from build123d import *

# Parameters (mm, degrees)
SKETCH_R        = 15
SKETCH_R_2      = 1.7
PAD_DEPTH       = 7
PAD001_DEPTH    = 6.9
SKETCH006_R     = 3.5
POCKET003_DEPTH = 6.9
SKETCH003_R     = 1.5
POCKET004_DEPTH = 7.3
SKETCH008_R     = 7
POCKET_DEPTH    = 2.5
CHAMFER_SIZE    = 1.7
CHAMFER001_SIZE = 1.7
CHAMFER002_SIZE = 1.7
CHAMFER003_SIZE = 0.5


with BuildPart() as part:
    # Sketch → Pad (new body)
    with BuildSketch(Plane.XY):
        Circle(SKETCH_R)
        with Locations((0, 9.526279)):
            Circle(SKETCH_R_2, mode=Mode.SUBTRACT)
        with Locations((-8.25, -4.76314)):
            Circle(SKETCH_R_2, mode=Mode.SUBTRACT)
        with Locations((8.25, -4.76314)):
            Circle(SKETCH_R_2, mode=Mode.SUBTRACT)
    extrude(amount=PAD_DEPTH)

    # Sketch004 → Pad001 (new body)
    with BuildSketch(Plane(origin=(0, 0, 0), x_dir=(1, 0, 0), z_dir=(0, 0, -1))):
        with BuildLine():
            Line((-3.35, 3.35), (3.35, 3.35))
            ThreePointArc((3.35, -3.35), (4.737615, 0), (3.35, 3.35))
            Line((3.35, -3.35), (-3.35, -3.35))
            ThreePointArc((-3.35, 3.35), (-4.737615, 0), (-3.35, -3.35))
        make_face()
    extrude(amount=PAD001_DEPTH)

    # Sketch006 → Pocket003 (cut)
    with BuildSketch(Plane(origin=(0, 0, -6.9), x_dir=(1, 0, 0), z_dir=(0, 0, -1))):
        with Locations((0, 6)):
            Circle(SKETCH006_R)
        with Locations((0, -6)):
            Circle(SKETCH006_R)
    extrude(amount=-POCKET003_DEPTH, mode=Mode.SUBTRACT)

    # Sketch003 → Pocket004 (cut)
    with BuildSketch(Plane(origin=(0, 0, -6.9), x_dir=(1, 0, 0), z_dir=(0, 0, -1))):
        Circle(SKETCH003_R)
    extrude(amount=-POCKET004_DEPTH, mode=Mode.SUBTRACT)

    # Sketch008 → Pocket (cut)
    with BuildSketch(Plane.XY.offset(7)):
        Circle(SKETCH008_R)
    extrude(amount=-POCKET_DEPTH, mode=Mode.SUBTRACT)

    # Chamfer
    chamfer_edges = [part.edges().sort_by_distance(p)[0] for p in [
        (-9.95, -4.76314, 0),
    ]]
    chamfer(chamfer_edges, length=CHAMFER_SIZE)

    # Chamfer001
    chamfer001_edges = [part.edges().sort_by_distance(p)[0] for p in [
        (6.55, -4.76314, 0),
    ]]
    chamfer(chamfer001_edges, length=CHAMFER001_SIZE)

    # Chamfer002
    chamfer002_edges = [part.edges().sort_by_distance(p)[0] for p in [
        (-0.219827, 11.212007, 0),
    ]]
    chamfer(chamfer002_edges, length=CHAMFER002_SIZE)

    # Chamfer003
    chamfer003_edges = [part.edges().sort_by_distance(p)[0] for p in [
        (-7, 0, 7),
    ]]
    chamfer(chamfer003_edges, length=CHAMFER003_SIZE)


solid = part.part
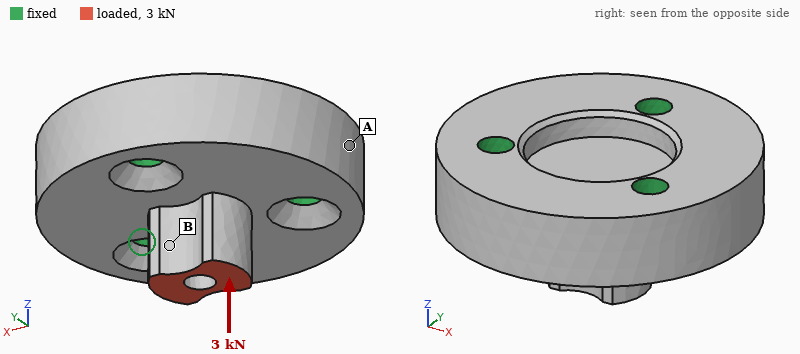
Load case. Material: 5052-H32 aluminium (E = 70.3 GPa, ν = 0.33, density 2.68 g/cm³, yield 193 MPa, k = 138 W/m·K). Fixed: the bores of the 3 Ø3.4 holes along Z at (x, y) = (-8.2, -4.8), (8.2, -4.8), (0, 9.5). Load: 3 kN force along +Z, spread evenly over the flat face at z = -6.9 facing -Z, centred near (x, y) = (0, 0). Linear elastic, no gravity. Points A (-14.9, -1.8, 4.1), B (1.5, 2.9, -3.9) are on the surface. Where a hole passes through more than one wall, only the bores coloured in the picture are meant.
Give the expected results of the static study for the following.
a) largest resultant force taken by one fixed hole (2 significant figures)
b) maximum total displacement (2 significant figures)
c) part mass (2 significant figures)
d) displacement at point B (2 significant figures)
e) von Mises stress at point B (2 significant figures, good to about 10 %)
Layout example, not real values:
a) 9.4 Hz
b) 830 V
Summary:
a) 1.1 kN
b) 15 µm
c) 12 g
d) 12 µm
e) 60 MPa
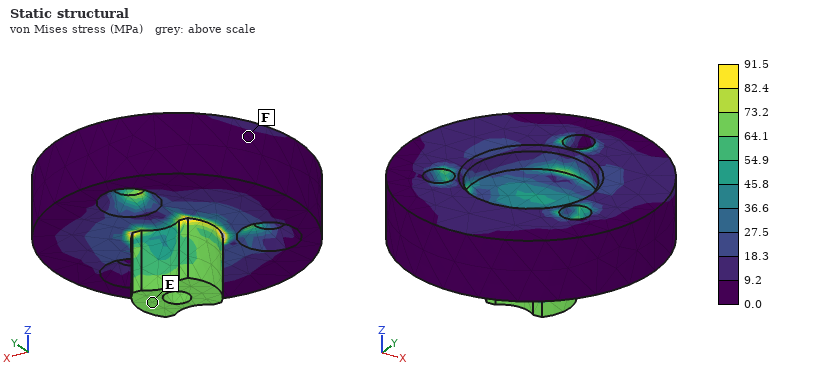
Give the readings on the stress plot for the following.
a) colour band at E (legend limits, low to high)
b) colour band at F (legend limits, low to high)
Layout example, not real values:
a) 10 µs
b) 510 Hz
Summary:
a) 64.1 to 73.2 MPa
b) 0.0 to 9.2 MPa
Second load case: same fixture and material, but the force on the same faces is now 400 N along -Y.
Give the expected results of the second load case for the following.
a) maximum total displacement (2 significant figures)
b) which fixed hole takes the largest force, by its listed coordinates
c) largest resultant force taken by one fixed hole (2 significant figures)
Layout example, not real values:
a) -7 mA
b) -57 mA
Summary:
a) 14 µm
b) (0, 9.5)
c) 320 N
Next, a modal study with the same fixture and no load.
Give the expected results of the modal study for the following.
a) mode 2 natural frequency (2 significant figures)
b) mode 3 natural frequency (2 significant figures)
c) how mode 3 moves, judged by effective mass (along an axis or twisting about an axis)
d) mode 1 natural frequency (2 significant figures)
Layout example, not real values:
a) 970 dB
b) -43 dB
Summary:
a) 38 kHz
b) 44 kHz
c) along Z
d) 38 kHz
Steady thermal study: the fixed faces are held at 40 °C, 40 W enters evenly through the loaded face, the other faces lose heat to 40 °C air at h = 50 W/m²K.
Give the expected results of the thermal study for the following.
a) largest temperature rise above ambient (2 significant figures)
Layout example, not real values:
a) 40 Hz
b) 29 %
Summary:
a) 61 K
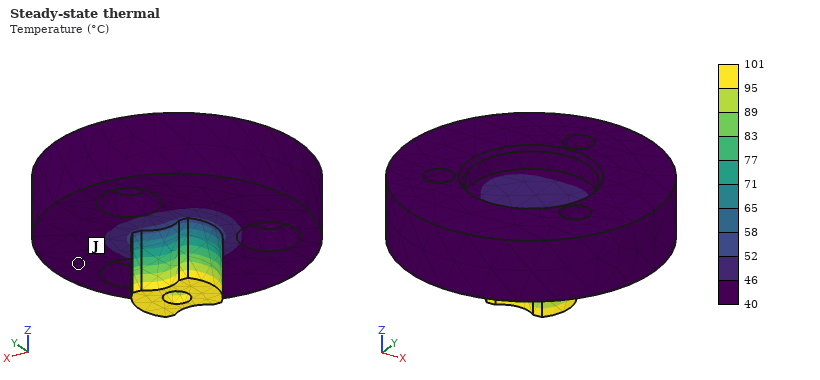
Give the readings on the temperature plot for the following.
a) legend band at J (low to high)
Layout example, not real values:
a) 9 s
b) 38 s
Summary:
a) 40 to 46 °C
